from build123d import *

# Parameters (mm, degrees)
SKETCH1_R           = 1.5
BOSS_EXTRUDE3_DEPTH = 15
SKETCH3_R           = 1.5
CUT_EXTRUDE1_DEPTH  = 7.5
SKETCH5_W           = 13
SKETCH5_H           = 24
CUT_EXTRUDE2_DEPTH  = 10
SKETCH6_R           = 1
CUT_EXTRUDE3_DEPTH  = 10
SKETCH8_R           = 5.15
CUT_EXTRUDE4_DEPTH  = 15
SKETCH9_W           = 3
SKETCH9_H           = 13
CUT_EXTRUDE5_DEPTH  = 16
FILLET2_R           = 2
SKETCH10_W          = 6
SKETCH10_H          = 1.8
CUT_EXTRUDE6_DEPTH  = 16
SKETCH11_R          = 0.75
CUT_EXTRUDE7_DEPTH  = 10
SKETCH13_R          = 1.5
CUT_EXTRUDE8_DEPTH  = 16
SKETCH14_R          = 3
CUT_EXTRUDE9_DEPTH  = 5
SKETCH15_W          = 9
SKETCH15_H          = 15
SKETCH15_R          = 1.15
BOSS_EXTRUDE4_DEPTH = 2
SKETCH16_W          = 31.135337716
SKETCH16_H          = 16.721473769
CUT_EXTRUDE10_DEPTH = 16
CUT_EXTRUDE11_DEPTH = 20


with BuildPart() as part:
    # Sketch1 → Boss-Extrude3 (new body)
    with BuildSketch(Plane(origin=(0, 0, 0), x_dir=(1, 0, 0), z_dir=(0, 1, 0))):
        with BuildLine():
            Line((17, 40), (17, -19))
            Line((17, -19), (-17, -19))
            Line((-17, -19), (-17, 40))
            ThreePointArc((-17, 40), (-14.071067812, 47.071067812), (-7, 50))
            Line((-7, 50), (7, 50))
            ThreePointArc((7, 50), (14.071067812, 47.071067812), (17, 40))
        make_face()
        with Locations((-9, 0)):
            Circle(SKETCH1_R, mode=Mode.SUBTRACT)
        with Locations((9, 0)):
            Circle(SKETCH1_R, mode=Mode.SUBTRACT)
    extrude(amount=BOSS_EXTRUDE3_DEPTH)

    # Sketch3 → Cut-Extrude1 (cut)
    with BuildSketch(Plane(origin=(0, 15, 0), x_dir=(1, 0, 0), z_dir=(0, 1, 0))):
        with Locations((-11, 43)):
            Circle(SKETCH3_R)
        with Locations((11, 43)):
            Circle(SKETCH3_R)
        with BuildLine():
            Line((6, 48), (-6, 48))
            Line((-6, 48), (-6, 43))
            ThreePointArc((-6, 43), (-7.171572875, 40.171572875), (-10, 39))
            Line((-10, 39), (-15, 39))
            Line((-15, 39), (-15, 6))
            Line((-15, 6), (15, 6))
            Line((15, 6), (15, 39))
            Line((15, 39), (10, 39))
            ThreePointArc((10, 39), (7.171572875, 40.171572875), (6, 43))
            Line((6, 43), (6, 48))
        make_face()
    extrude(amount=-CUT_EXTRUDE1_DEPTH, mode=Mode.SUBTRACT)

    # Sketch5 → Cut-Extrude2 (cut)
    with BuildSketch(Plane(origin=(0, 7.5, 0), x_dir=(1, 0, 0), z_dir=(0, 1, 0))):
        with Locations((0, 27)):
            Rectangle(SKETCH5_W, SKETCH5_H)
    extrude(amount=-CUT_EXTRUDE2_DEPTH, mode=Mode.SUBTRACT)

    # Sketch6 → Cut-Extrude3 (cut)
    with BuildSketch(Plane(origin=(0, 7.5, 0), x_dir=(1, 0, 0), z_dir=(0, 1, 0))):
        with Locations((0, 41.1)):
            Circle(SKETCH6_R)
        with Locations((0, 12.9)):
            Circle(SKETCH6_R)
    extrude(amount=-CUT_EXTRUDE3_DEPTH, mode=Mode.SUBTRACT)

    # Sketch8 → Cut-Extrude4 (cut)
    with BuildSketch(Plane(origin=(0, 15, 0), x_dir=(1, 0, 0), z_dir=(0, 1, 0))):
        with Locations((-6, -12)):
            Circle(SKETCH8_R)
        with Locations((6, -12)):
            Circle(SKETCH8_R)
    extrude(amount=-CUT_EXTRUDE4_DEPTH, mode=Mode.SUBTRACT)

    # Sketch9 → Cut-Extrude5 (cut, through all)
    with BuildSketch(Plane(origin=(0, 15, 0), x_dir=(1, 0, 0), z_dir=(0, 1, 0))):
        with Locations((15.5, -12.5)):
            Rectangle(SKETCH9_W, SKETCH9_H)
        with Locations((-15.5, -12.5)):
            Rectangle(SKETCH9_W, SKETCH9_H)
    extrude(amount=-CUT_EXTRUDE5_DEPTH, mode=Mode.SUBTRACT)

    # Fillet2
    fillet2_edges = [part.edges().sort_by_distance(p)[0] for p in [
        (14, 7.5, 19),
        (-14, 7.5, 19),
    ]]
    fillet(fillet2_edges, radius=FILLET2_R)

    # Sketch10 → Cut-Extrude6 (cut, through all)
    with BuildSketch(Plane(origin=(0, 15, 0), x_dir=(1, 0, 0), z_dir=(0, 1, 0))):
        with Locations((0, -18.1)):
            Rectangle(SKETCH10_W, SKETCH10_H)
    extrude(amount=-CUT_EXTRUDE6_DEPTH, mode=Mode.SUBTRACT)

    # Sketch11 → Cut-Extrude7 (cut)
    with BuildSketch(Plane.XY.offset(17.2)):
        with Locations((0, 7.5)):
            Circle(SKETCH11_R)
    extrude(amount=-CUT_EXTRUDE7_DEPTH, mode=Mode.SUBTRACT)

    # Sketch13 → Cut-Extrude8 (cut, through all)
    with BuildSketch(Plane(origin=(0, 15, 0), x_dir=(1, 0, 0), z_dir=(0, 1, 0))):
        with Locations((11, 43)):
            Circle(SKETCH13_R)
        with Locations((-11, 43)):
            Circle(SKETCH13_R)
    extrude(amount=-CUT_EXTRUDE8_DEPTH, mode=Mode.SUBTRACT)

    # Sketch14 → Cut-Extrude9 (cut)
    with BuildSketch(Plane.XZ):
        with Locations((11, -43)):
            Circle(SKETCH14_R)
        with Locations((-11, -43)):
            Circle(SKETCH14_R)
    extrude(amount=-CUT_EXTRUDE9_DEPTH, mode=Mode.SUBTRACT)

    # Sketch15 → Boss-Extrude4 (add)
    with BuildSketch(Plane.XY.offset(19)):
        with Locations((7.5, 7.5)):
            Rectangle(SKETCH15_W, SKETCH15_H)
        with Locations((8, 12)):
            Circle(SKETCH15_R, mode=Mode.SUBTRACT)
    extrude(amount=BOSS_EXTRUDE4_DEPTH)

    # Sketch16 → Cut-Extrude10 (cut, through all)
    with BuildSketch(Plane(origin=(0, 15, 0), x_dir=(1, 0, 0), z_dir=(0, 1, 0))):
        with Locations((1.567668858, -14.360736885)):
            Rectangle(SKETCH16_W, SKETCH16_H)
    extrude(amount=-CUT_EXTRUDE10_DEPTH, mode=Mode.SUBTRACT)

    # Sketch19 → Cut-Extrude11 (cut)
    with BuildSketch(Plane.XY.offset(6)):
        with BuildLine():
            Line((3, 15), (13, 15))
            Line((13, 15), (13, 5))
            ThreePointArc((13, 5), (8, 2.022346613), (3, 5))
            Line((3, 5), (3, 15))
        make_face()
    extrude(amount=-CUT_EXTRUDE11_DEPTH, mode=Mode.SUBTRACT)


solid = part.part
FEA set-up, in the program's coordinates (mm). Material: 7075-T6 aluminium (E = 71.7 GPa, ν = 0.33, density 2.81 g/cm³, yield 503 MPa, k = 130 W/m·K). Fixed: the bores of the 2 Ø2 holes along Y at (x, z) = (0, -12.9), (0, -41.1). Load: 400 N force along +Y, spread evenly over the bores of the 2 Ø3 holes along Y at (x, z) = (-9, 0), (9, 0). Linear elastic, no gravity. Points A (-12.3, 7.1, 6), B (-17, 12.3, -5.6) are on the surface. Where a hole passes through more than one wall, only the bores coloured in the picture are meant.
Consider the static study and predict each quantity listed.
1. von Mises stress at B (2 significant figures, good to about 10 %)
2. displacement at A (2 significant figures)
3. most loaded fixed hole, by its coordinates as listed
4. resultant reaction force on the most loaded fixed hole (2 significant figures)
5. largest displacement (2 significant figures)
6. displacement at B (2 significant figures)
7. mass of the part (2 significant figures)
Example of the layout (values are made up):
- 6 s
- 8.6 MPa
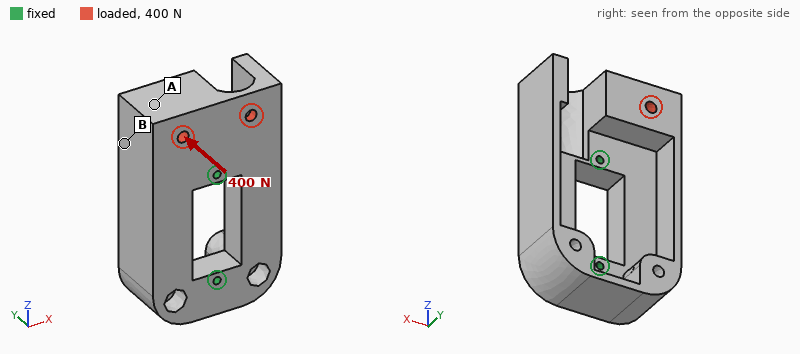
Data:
- 6.6 MPa
- 22 µm
- (0, -12.9)
- 470 N
- 27 µm
- 18 µm
- 42 g
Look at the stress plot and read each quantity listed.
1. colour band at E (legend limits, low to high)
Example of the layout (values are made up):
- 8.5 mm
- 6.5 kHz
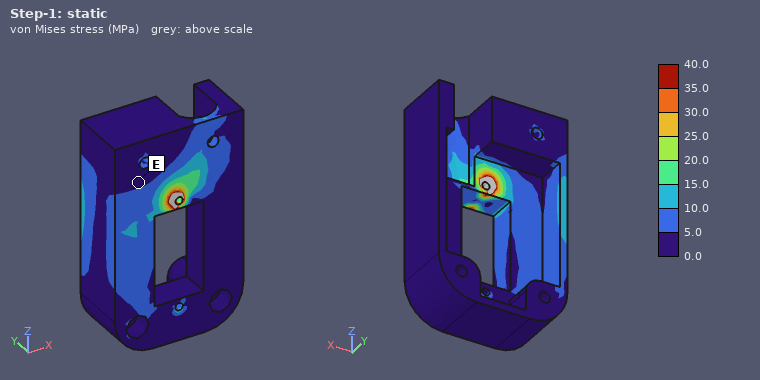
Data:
- 0.0 to 5.0 MPa
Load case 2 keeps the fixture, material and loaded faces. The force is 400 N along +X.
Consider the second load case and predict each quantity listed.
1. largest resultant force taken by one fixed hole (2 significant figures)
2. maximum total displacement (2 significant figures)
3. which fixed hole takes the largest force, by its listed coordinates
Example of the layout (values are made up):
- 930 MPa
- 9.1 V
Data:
- 540 N
- 13 µm
- (0, -12.9)
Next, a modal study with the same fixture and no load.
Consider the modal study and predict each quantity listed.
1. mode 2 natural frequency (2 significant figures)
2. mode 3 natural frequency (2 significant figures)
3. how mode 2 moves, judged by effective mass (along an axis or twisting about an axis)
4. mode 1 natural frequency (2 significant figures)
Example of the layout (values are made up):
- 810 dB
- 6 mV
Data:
- 6800 Hz
- 8700 Hz
- along Y
- 5700 Hz
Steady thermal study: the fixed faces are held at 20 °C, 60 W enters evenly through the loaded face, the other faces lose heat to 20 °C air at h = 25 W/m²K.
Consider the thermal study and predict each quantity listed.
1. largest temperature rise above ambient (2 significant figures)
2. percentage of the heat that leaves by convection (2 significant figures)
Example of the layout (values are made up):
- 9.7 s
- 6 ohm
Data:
- 52 K
- 6.0 %
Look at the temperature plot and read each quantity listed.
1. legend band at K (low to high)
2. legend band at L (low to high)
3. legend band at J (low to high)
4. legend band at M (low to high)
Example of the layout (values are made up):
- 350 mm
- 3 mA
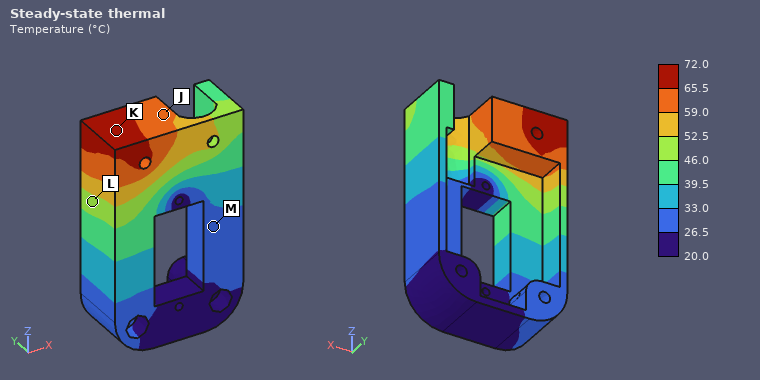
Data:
- 65.5 to 72.0 °C
- 46.0 to 52.5 °C
- 59.0 to 65.5 °C
- 26.5 to 33.0 °C
